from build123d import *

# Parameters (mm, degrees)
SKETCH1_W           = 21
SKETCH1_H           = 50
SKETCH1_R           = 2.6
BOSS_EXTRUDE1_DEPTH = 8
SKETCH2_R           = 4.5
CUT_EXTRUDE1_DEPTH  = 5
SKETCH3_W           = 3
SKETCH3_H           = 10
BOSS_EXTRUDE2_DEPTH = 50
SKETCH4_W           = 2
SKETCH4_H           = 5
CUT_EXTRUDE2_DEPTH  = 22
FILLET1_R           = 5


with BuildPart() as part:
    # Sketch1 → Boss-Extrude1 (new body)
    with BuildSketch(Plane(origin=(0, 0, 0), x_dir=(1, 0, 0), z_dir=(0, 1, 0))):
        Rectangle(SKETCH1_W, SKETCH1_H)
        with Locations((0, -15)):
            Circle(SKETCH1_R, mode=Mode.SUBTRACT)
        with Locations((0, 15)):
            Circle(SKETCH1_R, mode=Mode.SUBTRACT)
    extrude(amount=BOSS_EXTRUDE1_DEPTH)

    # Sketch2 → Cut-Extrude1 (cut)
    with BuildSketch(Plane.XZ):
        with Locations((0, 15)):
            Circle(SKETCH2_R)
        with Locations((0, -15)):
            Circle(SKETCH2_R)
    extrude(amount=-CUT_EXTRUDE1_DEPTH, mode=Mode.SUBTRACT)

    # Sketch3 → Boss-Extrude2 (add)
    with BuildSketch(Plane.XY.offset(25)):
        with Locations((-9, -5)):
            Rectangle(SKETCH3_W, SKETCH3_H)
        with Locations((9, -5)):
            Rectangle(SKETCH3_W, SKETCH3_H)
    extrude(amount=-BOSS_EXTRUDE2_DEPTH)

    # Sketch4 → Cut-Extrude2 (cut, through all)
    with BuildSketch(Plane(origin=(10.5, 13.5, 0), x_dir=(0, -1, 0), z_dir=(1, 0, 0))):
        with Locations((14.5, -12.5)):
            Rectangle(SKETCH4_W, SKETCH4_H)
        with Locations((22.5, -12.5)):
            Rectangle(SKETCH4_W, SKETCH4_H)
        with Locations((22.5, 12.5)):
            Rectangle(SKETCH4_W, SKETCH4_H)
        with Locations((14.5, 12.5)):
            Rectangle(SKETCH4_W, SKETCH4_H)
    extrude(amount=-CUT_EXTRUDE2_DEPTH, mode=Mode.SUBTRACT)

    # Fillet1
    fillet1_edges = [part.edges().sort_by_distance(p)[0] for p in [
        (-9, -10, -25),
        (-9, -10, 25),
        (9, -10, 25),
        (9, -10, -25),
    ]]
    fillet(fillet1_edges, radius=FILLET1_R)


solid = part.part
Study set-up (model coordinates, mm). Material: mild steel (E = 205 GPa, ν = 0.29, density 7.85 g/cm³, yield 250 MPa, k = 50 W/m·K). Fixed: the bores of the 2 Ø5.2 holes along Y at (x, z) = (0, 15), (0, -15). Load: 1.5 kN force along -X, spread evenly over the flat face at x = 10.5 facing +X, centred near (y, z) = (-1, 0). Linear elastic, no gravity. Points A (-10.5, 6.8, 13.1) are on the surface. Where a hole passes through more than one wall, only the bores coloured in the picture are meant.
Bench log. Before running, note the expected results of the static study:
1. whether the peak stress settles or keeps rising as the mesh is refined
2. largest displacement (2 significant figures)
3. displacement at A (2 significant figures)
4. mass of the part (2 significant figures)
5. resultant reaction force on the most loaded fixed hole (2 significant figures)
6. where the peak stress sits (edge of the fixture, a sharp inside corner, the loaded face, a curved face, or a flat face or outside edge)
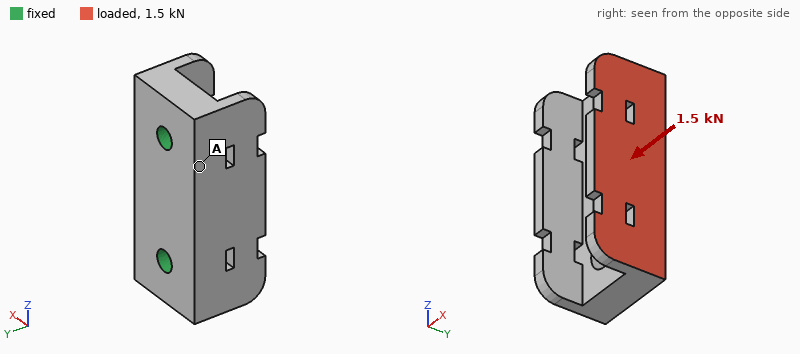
keeps rising
23 µm
5.3 µm
81 g
750 N
edge of the fixture
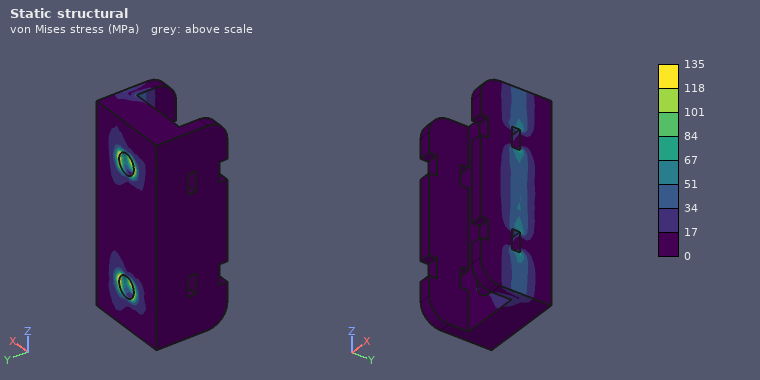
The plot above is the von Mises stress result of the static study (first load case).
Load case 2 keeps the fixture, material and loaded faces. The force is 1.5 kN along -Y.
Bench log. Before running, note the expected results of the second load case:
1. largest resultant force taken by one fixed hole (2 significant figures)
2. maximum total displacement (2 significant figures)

760 N
21 µm
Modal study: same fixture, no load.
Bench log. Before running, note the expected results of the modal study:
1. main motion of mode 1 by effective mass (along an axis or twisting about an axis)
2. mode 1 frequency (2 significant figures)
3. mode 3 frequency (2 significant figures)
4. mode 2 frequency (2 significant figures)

along X
7700 Hz
16 kHz
13 kHz
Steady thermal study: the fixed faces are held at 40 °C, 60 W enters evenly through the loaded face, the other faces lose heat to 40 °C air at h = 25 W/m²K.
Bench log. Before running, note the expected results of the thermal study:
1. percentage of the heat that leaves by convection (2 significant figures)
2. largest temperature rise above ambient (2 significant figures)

6.5 %
86 K
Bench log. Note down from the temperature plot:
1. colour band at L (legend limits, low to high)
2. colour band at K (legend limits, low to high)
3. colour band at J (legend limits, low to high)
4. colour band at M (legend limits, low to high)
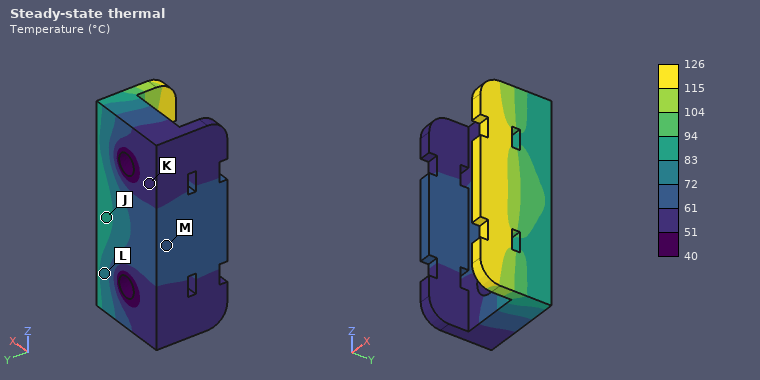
72 to 83 °C
51 to 61 °C
83 to 94 °C
61 to 72 °C
